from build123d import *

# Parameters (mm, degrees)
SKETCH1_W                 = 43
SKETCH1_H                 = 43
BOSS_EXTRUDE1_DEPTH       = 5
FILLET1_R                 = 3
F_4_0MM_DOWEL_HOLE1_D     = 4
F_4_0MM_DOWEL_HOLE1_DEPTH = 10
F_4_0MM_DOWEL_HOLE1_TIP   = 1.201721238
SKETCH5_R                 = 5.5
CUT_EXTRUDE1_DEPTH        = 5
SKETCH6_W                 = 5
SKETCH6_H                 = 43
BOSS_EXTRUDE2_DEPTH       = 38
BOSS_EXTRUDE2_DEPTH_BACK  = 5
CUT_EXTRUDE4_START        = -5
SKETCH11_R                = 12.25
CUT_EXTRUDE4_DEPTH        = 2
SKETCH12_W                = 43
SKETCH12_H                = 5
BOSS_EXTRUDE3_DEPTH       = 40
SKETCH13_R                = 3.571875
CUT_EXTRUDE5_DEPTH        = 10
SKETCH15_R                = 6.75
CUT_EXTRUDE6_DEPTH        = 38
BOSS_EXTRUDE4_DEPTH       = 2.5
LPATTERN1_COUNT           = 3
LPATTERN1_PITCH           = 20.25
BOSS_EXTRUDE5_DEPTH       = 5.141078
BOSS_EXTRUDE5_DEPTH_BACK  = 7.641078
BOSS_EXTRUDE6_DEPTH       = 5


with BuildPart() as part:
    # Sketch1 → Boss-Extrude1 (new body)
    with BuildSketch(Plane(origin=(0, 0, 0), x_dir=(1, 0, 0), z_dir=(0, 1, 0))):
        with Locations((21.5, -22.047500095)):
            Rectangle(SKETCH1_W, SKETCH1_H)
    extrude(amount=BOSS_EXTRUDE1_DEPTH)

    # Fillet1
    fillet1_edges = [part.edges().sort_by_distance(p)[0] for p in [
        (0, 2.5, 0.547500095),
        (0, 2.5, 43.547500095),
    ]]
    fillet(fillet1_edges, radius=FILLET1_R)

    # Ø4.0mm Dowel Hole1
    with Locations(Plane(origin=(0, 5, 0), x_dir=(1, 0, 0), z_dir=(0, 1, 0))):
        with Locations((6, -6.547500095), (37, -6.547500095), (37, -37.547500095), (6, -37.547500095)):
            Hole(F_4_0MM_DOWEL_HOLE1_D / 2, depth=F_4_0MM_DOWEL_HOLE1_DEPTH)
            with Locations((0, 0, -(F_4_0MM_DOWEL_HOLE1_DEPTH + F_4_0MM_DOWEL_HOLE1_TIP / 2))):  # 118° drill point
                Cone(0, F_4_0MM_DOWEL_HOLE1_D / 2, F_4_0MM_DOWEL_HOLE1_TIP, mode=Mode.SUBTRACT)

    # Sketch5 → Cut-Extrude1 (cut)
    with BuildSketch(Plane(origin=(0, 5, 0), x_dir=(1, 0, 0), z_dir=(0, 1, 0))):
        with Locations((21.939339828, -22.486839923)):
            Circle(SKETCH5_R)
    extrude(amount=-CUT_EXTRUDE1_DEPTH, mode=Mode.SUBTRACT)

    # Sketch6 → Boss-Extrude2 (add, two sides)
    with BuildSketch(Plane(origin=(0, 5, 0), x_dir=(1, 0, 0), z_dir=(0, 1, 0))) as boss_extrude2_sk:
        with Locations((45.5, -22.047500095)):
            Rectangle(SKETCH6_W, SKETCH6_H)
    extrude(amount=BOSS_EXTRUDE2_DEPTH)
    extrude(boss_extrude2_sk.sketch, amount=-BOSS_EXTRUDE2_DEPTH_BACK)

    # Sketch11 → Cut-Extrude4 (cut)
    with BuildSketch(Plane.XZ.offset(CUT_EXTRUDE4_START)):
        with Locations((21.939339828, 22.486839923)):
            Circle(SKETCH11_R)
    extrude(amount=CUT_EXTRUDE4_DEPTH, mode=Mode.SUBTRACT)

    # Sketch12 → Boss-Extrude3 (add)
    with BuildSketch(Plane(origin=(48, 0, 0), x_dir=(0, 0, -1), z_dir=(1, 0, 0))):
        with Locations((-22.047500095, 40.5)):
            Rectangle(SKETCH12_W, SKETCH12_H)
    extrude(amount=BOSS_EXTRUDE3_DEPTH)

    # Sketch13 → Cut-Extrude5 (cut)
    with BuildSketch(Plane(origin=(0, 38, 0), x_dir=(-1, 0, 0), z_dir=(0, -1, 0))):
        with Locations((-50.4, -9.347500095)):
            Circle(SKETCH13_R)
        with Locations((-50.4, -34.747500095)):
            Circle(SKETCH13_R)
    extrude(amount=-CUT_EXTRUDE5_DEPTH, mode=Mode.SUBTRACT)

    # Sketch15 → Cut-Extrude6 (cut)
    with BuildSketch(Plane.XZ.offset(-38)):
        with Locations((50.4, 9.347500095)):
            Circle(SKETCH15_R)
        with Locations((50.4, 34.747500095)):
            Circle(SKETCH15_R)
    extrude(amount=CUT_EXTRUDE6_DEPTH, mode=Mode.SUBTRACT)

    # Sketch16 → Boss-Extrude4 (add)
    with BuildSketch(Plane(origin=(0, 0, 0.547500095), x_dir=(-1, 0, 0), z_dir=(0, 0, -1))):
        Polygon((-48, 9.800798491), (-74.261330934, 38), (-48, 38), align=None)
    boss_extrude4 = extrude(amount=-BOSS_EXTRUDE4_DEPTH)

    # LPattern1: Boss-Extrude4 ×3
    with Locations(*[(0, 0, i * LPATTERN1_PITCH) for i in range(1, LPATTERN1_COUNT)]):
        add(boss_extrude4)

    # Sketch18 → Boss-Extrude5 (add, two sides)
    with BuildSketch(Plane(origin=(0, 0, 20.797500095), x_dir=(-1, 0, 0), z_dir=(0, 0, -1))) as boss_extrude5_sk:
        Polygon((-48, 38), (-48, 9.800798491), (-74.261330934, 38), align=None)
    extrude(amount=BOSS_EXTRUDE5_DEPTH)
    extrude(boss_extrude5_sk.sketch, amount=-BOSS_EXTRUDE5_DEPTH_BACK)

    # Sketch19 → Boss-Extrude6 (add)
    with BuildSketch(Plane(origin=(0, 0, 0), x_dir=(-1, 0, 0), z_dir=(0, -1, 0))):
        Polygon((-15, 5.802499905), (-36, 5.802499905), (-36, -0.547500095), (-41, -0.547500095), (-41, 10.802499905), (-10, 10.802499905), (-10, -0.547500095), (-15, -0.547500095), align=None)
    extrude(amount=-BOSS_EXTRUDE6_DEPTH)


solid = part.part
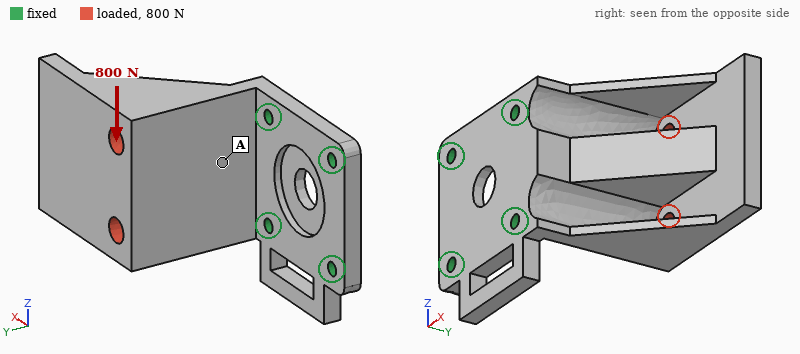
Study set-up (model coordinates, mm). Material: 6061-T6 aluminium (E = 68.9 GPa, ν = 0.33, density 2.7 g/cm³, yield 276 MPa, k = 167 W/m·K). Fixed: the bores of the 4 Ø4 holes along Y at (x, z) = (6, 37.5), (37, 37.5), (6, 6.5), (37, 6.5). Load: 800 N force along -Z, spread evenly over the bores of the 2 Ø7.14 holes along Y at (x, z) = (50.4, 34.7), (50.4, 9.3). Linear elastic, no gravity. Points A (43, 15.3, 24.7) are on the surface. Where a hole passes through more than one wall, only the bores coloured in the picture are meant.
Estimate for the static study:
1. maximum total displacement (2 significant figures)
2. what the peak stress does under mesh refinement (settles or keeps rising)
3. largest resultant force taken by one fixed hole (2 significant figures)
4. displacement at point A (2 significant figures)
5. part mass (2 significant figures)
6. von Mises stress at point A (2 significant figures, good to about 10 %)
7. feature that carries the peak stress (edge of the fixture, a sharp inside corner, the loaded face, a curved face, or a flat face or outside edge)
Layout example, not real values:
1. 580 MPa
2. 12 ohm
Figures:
1. 55 µm
2. keeps rising
3. 1.1 kN
4. 15 µm
5. 81 g
6. 9.5 MPa
7. edge of the fixture
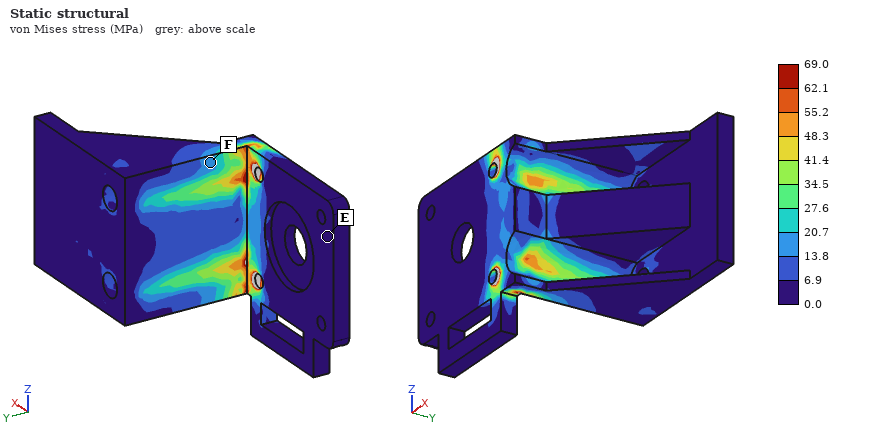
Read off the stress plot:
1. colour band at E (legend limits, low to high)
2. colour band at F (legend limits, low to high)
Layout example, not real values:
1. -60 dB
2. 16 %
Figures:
1. 0.0 to 6.9 MPa
2. 13.8 to 20.7 MPa
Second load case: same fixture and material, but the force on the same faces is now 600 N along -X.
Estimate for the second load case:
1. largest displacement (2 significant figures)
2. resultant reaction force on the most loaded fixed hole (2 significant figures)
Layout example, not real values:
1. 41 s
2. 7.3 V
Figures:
1. 1.1 mm
2. 350 N
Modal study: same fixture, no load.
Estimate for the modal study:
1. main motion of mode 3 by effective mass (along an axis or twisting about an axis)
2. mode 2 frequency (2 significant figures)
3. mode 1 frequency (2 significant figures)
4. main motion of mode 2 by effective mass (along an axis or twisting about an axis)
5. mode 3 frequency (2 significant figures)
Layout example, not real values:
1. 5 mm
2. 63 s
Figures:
1. along Z
2. 2200 Hz
3. 650 Hz
4. along Z
5. 4000 Hz
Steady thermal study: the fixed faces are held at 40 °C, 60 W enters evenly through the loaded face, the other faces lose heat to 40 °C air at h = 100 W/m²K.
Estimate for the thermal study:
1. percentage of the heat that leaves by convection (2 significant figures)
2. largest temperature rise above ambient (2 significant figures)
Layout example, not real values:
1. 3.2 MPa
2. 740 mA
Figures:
1. 54 %
2. 47 K
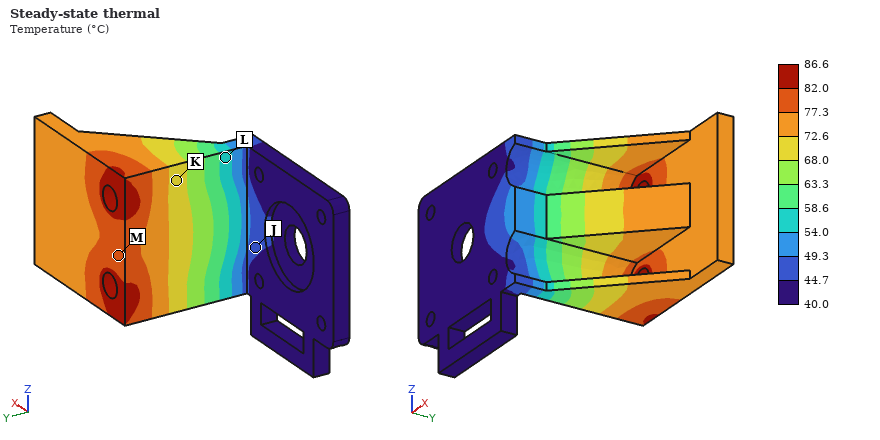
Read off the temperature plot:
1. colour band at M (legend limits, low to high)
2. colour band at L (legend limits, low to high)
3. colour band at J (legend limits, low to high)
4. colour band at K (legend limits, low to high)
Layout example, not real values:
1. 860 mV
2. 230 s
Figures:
1. 77.3 to 82.0 °C
2. 54.0 to 58.6 °C
3. 44.7 to 49.3 °C
4. 68.0 to 72.6 °C
